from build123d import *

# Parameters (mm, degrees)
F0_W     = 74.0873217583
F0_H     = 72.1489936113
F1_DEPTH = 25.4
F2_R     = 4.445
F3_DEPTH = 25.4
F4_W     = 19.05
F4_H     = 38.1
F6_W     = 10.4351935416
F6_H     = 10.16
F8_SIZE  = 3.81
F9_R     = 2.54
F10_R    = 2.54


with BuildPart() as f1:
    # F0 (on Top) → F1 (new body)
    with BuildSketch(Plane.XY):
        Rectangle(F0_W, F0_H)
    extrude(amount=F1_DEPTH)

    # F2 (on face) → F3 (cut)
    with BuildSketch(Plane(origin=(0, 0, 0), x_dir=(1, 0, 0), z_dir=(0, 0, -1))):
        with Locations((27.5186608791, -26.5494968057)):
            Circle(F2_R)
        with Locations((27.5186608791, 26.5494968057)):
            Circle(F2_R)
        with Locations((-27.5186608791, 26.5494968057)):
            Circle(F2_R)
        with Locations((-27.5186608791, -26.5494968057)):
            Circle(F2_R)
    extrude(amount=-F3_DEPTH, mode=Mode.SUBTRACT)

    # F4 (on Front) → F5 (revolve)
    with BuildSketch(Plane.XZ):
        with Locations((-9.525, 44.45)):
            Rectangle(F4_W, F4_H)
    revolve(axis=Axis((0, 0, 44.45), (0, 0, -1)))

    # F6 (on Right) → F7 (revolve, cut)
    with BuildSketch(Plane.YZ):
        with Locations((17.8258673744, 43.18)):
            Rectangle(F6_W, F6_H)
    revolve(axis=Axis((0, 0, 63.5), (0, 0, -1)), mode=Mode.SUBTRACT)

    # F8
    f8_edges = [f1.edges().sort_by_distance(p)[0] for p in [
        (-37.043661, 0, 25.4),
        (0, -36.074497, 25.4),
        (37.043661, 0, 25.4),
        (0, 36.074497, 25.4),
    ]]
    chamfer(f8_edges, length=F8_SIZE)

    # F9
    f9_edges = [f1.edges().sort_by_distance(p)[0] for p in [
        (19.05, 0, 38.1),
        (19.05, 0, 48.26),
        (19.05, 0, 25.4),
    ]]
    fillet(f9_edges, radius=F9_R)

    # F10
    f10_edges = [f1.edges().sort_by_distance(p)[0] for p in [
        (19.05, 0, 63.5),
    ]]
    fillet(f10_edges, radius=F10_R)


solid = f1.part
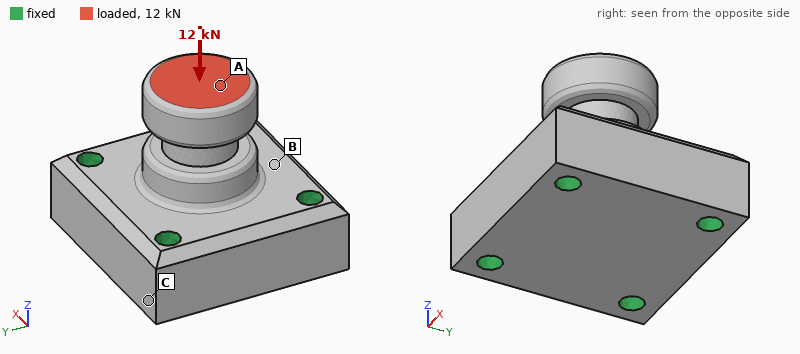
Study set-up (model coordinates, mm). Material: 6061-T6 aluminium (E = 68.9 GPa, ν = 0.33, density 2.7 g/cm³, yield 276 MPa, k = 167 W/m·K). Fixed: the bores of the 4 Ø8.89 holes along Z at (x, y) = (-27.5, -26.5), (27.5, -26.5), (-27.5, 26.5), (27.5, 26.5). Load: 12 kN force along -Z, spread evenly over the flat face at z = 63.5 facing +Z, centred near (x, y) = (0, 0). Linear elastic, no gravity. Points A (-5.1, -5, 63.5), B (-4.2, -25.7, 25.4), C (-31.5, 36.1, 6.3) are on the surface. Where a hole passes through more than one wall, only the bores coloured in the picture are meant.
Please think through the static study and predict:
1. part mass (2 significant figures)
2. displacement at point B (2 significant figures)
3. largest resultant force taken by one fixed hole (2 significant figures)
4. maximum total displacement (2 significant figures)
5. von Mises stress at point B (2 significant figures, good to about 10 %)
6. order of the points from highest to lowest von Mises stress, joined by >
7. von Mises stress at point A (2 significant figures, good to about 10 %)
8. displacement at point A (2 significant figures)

440 g
3.2 µm
3.1 kN
16 µm
4.3 MPa
A > B > C
16 MPa
15 µm
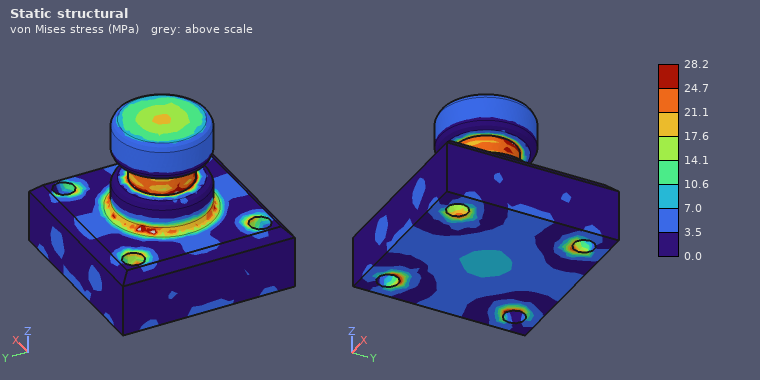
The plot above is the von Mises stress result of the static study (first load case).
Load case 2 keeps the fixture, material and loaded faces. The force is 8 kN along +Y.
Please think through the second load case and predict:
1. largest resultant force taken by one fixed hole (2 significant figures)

4.5 kN
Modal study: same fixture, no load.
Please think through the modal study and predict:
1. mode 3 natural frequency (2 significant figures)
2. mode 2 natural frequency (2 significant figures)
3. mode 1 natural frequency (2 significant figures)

13 kHz
8000 Hz
8000 Hz
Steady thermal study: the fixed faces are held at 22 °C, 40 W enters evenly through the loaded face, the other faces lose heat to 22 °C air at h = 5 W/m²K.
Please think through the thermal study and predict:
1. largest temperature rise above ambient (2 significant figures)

16 K
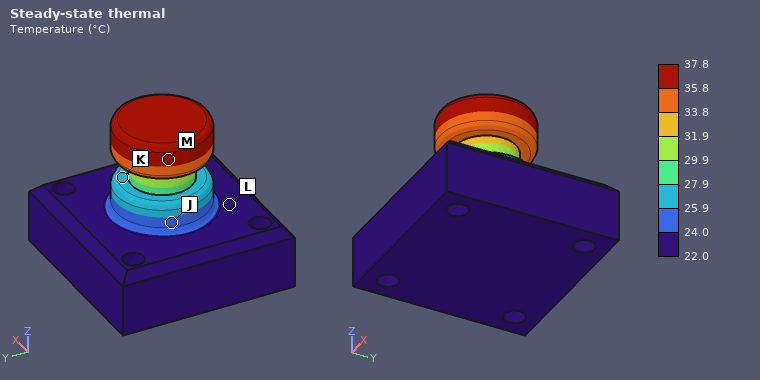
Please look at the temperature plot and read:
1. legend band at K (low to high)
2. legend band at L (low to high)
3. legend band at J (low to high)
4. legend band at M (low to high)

25.9 to 27.9 °C
22.0 to 24.0 °C
24.0 to 25.9 °C
35.8 to 37.8 °C
